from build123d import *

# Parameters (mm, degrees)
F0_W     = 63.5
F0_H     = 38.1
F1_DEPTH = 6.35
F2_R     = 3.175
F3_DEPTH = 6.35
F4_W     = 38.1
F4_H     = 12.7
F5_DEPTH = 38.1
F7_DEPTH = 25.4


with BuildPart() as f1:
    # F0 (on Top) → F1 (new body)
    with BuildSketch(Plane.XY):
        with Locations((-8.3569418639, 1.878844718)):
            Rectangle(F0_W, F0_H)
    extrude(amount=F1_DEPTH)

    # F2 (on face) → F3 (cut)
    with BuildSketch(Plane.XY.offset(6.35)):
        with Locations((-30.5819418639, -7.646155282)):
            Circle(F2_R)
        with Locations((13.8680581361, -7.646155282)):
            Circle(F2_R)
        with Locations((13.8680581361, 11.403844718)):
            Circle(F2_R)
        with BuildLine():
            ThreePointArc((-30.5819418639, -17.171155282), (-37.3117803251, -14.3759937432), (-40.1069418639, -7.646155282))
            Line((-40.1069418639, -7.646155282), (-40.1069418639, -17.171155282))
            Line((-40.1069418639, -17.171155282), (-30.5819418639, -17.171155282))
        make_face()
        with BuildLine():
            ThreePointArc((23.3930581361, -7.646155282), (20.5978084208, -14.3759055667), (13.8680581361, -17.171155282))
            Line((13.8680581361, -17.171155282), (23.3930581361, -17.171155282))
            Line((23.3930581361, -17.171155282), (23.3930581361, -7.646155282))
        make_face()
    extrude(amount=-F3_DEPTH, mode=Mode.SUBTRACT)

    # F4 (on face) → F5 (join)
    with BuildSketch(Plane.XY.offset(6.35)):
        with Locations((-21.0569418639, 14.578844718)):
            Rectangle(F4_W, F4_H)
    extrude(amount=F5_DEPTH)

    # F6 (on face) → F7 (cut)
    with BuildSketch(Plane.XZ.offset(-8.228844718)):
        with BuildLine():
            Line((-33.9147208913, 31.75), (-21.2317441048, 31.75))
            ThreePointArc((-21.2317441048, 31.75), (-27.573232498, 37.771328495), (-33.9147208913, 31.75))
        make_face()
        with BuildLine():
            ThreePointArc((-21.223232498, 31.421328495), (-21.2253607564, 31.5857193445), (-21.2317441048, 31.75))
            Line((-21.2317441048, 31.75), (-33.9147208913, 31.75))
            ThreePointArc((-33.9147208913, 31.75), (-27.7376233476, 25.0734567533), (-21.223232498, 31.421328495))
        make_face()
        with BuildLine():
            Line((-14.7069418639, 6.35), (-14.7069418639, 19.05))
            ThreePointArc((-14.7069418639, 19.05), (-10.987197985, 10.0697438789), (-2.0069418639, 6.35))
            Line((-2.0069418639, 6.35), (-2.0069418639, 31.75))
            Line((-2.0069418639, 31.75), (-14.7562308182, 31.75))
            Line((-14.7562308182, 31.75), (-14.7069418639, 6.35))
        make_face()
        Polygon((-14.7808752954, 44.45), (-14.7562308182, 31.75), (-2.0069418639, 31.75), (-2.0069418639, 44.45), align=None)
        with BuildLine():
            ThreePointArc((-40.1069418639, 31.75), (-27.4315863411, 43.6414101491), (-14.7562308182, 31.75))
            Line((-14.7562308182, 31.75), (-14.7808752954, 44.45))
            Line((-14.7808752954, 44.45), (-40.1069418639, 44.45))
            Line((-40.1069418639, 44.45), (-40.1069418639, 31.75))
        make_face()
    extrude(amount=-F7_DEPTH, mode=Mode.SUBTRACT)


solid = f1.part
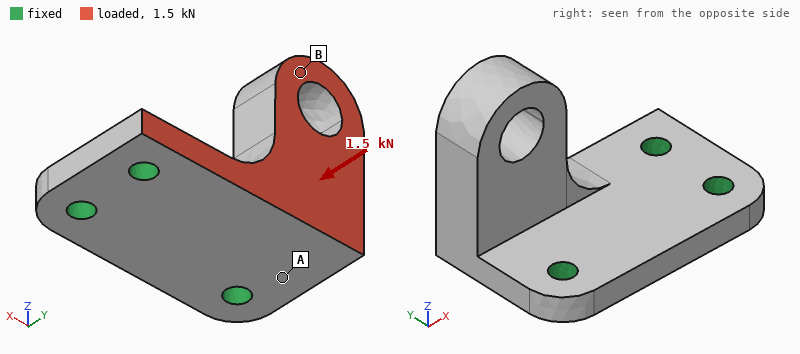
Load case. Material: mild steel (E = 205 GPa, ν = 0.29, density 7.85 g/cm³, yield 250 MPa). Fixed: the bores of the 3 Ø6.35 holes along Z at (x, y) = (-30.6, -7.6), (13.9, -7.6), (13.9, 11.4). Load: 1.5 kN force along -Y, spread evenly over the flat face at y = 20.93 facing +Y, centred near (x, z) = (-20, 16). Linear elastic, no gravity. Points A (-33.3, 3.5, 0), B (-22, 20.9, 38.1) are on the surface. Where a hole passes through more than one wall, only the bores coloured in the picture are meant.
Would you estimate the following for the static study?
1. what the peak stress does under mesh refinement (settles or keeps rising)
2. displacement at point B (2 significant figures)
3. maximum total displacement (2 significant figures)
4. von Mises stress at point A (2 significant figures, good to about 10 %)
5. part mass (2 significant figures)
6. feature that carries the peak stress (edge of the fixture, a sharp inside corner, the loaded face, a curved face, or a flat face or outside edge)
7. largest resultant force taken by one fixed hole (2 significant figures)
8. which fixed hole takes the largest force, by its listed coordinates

keeps rising
61 µm
71 µm
45 MPa
190 g
edge of the fixture
1.0 kN
(-30.6, -7.6)
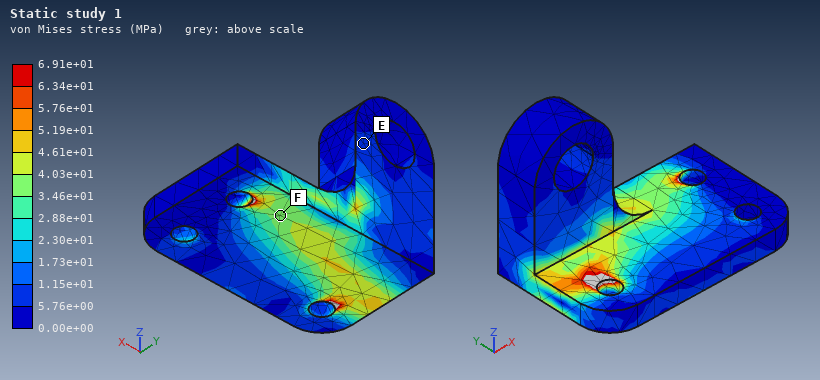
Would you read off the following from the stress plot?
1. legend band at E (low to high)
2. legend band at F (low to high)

5.76e+00 to 1.15e+01 MPa
3.46e+01 to 4.03e+01 MPa
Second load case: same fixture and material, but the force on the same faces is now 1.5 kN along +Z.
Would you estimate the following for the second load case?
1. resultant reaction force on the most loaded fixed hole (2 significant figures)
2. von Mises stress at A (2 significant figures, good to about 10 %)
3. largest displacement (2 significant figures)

950 N
58 MPa
86 µm
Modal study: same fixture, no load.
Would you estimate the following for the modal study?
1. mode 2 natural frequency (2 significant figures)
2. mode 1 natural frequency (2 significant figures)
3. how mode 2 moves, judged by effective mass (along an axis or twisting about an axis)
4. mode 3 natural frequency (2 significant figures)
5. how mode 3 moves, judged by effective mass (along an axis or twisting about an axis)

4400 Hz
2400 Hz
along X
7500 Hz
along Z
